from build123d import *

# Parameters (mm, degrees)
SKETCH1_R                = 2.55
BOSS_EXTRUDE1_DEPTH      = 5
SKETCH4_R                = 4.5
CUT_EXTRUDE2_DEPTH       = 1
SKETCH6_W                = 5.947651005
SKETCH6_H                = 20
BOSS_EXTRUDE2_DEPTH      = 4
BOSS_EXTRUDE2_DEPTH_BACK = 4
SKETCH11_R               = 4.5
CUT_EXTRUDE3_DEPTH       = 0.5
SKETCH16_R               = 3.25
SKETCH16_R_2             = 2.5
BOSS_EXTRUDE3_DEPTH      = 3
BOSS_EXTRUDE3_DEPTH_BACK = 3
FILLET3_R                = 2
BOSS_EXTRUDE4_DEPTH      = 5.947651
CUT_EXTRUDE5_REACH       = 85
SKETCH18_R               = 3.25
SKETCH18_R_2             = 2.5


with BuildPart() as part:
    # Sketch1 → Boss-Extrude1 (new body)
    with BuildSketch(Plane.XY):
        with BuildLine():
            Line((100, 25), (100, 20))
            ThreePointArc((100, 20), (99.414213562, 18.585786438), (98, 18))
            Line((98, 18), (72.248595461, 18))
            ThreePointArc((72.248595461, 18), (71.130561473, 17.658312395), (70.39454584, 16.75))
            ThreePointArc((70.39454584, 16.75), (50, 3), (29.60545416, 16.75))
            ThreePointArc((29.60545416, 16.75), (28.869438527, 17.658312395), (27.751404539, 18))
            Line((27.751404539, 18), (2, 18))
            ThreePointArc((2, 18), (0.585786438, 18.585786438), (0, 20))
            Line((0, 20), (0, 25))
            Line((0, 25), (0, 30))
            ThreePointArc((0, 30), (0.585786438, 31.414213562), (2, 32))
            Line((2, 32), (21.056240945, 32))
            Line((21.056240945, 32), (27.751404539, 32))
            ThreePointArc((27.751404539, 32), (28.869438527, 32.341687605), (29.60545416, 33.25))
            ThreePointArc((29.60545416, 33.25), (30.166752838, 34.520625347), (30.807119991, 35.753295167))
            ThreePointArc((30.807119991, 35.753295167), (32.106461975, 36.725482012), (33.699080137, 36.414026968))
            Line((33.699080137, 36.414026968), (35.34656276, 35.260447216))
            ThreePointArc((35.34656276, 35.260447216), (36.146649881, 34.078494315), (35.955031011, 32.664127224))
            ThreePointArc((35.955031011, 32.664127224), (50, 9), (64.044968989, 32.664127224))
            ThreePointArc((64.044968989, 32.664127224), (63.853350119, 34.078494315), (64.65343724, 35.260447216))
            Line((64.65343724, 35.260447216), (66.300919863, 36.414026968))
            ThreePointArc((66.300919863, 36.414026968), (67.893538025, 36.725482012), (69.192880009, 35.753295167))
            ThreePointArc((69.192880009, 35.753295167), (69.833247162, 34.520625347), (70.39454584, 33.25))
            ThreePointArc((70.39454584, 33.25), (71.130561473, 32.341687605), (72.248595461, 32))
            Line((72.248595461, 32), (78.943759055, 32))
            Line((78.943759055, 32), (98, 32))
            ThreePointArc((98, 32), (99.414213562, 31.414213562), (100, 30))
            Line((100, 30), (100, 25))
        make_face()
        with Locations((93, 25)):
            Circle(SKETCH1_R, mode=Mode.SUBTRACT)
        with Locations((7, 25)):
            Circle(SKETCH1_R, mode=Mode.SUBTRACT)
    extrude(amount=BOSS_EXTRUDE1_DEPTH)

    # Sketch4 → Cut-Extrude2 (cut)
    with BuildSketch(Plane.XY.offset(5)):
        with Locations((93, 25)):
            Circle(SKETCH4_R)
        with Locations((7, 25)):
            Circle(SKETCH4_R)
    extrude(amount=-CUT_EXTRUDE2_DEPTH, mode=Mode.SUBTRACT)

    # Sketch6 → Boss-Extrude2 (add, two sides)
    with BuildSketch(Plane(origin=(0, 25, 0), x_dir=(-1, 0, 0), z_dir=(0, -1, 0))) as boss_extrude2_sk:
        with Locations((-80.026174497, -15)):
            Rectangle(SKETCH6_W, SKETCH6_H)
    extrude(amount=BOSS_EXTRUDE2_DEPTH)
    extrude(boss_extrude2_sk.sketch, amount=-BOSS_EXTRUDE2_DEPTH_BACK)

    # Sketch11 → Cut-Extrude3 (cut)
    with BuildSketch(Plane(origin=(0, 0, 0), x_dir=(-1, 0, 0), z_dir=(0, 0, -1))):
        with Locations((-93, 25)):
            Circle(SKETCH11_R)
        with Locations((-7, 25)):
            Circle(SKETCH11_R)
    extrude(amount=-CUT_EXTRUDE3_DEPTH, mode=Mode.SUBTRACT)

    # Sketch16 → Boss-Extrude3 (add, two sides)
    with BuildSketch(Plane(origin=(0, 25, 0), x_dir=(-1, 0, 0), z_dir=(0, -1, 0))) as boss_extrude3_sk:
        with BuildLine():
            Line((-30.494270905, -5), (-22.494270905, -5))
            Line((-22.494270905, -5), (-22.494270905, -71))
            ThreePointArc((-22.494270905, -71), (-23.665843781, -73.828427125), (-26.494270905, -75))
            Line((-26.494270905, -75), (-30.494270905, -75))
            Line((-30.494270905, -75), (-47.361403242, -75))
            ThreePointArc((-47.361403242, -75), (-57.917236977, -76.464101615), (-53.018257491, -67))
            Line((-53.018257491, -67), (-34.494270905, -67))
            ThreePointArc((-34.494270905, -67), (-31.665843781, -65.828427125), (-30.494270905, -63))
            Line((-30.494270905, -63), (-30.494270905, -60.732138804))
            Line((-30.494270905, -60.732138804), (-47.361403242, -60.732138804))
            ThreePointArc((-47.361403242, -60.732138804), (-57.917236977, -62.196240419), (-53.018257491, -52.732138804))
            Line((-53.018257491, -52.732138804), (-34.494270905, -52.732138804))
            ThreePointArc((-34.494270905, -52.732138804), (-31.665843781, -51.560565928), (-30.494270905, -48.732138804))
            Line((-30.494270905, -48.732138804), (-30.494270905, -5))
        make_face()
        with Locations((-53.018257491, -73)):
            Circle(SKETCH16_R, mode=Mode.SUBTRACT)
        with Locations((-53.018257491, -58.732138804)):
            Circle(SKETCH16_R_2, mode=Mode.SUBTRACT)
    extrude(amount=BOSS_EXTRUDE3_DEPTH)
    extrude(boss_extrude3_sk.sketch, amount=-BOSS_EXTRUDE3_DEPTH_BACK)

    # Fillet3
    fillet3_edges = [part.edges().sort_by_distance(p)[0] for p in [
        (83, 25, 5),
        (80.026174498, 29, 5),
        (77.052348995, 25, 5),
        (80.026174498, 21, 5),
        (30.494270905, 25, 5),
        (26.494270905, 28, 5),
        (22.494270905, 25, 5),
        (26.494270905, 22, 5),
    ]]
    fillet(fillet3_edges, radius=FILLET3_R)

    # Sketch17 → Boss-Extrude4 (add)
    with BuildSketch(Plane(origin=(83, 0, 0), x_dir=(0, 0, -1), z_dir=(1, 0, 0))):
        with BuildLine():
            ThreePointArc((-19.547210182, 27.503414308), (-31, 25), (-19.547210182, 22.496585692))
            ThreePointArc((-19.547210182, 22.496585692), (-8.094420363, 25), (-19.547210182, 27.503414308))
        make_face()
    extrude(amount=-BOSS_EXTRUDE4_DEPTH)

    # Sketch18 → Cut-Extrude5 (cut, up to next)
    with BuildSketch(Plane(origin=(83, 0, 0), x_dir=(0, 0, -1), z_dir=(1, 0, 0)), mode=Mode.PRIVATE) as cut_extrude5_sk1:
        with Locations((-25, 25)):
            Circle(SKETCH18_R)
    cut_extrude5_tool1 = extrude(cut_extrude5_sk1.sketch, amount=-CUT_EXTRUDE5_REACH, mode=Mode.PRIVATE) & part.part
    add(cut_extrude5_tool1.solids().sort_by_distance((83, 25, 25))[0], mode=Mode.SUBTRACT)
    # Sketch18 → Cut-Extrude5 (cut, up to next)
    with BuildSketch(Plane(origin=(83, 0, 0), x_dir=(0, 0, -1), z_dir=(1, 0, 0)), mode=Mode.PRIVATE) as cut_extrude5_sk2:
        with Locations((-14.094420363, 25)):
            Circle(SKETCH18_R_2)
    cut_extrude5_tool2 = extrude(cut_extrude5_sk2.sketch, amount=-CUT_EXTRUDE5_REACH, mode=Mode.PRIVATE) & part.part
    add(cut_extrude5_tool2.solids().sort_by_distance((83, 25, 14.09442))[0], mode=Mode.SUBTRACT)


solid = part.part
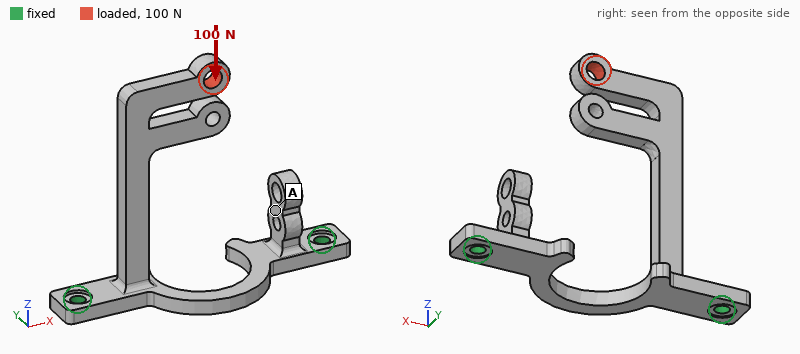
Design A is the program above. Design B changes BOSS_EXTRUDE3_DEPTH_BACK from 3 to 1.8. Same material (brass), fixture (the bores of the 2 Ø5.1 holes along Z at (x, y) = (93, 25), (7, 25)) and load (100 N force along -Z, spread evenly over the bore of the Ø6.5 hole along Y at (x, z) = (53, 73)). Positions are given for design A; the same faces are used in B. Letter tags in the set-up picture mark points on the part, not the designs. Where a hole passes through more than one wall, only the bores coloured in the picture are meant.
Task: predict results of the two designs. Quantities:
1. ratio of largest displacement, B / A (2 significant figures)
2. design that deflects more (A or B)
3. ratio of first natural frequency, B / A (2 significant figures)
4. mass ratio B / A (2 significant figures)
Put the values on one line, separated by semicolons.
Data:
1.1; B; 0.90; 0.91
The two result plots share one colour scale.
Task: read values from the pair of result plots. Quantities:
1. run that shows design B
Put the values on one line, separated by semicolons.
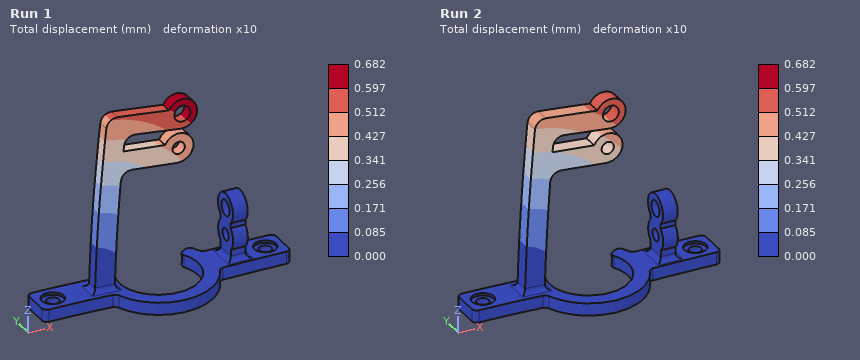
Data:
Run 1
